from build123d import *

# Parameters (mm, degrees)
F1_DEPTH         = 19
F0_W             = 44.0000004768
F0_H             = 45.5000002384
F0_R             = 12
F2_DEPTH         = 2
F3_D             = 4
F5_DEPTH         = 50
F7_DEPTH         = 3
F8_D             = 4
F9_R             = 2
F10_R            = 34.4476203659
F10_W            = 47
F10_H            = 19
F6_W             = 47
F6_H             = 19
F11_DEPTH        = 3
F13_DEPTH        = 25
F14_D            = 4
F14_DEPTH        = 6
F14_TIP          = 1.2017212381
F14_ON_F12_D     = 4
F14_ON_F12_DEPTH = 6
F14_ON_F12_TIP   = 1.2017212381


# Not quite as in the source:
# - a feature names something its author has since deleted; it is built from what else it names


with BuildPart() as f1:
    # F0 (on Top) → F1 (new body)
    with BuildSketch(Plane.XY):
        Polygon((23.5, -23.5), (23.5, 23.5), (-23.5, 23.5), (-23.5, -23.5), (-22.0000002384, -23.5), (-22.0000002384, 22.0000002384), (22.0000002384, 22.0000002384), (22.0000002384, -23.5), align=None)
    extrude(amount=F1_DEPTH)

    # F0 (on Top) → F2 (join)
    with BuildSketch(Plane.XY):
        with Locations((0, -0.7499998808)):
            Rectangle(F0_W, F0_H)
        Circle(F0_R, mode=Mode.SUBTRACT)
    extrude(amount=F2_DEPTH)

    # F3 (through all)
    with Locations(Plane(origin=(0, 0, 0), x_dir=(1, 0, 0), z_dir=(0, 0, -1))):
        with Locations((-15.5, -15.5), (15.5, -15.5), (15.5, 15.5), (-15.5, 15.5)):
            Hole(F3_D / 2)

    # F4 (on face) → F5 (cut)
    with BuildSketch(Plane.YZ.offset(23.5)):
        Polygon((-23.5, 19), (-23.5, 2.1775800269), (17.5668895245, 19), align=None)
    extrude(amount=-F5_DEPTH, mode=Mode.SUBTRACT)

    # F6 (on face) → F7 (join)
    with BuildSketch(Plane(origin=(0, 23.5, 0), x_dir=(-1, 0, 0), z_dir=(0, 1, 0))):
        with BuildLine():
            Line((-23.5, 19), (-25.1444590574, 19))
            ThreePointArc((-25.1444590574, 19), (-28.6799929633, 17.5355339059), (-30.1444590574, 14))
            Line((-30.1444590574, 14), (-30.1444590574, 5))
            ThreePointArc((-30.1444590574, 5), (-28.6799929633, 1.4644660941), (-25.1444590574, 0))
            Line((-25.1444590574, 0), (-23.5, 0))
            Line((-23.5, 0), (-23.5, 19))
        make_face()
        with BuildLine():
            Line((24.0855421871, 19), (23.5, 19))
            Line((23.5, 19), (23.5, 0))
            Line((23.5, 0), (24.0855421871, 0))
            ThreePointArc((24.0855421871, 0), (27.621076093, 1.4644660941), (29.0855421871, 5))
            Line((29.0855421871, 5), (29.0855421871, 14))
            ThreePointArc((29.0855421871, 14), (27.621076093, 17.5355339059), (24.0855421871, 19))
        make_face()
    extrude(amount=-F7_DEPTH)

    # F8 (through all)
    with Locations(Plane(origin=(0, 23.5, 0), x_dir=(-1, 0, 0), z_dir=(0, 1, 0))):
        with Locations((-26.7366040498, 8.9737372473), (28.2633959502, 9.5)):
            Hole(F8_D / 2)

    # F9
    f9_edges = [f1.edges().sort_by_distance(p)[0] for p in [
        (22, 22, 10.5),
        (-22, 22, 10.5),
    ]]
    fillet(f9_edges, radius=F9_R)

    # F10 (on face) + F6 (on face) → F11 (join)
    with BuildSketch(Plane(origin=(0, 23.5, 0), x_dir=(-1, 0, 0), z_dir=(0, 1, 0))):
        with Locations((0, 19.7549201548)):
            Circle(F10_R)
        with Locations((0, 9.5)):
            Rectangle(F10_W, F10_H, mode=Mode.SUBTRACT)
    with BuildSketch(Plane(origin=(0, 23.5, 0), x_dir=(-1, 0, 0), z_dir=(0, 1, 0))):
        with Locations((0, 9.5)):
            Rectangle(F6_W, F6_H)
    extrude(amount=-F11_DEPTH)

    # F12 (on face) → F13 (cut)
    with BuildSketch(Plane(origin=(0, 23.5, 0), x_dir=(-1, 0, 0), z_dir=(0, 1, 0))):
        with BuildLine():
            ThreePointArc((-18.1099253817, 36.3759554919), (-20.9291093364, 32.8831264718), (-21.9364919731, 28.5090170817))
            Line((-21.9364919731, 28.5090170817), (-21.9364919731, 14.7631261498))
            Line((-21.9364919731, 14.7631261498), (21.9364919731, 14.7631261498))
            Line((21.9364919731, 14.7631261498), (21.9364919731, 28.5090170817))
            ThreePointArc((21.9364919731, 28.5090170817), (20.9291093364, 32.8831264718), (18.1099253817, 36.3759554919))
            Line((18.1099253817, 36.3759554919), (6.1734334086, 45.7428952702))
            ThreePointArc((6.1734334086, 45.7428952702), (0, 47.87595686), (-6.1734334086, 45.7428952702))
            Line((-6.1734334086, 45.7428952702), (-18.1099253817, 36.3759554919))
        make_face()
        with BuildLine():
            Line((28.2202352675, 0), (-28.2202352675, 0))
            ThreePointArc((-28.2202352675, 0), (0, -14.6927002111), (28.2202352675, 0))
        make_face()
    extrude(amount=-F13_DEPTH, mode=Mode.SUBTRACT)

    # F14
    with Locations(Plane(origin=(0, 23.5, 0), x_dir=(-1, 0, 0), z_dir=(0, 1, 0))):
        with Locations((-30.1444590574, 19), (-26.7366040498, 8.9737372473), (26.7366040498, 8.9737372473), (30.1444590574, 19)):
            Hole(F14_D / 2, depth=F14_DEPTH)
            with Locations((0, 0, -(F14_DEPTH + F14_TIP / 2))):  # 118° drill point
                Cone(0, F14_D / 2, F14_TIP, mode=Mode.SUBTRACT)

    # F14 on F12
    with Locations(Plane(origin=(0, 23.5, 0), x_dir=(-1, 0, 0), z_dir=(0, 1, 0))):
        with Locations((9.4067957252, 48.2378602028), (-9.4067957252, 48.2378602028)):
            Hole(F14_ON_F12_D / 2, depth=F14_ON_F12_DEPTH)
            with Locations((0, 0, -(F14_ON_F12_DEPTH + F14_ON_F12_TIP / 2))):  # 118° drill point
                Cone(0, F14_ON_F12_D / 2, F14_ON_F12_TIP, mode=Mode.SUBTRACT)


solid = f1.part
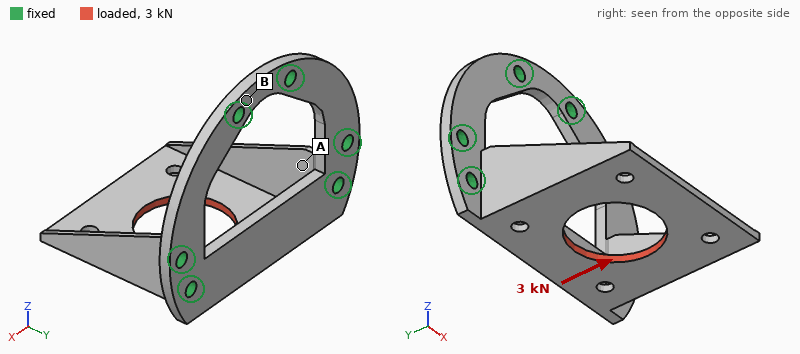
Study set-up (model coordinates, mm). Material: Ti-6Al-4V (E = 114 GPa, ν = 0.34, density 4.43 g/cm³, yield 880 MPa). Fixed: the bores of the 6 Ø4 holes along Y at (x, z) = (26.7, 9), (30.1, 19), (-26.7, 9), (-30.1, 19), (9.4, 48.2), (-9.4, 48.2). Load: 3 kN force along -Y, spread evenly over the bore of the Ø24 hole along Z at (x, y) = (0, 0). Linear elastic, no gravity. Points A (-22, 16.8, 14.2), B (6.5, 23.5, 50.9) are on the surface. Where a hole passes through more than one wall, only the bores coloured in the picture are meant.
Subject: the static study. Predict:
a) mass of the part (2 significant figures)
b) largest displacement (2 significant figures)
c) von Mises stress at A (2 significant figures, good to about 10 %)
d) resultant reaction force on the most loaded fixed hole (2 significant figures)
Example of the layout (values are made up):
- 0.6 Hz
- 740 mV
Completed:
- 44 g
- 0.23 mm
- 55 MPa
- 2.1 kN
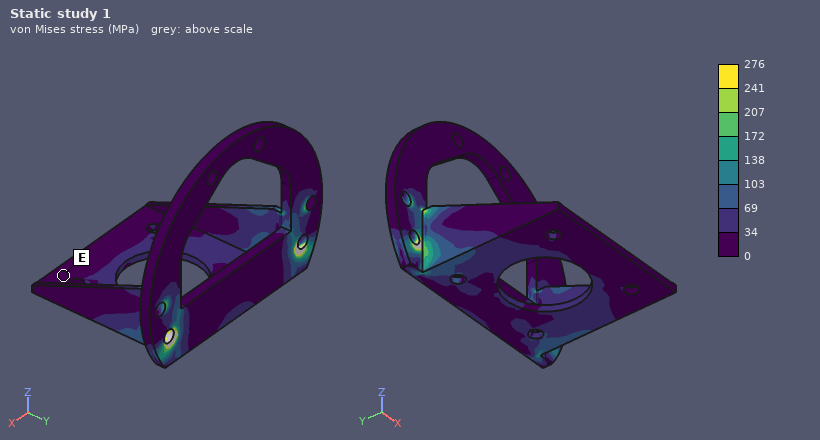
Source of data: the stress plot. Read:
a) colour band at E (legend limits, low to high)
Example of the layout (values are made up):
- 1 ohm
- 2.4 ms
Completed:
- 0 to 34 MPa
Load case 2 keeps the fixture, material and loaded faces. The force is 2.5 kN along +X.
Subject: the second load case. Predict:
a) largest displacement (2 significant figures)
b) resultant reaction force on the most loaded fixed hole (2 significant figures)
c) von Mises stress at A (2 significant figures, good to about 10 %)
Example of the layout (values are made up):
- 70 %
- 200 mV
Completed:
- 0.17 mm
- 1.9 kN
- 59 MPa
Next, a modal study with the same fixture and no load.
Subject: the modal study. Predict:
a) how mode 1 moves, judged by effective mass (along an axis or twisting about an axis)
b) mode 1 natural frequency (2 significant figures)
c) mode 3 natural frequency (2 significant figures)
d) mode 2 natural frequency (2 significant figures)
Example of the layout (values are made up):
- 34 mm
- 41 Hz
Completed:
- along Z
- 2300 Hz
- 5900 Hz
- 4100 Hz
